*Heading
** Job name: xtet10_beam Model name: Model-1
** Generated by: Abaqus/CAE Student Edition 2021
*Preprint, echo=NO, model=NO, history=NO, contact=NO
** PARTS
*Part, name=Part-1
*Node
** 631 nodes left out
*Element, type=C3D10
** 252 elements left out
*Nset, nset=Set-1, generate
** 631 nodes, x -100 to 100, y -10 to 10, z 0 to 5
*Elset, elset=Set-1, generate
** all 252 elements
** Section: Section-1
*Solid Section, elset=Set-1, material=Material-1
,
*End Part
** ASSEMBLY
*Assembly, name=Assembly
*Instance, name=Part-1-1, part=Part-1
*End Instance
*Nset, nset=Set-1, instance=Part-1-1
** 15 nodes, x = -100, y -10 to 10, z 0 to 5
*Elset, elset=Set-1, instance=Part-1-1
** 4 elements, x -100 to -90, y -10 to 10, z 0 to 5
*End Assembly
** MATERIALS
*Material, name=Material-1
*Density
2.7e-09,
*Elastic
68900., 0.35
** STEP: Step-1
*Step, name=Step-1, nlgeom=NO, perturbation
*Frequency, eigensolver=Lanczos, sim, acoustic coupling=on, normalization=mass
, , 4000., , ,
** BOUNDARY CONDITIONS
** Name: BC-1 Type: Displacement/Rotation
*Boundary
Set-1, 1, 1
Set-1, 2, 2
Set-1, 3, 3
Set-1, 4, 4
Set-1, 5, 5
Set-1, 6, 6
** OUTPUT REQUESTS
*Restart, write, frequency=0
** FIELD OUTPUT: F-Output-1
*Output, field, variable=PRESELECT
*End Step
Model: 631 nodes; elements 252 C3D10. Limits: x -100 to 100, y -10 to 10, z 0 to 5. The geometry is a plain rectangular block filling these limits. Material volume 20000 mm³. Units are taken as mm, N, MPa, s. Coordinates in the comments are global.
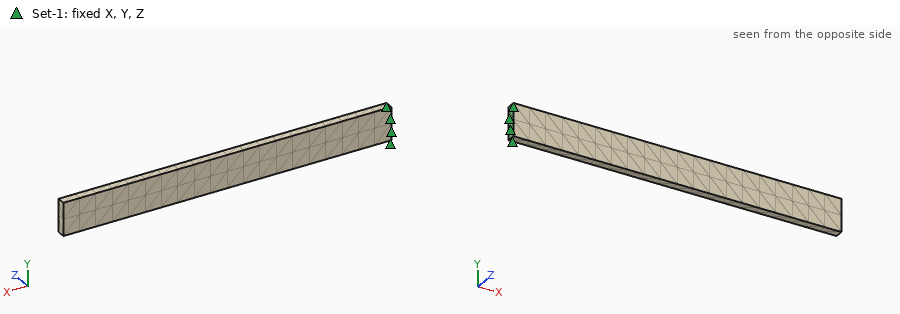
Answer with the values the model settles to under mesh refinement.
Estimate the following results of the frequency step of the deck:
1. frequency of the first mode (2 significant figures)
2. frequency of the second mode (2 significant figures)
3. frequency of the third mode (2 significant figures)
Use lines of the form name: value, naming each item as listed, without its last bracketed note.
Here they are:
frequency of the first mode: 100 Hz
frequency of the second mode: 410 Hz
frequency of the third mode: 640 Hz
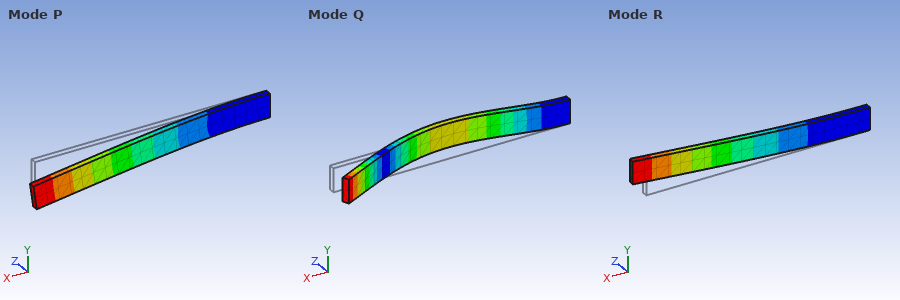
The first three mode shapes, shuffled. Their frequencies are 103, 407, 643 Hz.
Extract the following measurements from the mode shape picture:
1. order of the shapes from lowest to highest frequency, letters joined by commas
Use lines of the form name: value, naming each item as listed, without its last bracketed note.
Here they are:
order of the shapes from lowest to highest frequency, letters joined by commas: R, P, Q
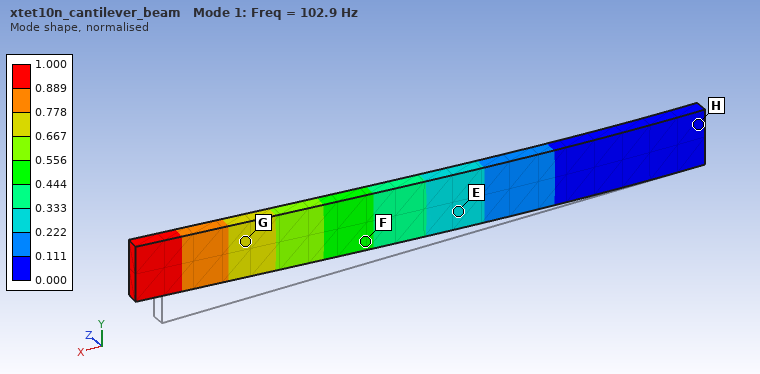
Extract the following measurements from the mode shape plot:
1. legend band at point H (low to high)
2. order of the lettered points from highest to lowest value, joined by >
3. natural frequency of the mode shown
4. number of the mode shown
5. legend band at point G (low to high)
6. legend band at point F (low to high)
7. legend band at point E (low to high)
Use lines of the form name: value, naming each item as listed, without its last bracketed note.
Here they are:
legend band at point H: 0.000 to 0.111
order of the lettered points from highest to lowest value, joined by >: G > F > E > H
natural frequency of the mode shown: 102.9 Hz
number of the mode shown: 1
legend band at point G: 0.667 to 0.778
legend band at point F: 0.444 to 0.556
legend band at point E: 0.222 to 0.333
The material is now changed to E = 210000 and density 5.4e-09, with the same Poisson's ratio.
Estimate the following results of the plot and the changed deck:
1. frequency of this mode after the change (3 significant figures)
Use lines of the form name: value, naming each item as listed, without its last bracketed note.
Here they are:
frequency of this mode after the change: 127 Hz
